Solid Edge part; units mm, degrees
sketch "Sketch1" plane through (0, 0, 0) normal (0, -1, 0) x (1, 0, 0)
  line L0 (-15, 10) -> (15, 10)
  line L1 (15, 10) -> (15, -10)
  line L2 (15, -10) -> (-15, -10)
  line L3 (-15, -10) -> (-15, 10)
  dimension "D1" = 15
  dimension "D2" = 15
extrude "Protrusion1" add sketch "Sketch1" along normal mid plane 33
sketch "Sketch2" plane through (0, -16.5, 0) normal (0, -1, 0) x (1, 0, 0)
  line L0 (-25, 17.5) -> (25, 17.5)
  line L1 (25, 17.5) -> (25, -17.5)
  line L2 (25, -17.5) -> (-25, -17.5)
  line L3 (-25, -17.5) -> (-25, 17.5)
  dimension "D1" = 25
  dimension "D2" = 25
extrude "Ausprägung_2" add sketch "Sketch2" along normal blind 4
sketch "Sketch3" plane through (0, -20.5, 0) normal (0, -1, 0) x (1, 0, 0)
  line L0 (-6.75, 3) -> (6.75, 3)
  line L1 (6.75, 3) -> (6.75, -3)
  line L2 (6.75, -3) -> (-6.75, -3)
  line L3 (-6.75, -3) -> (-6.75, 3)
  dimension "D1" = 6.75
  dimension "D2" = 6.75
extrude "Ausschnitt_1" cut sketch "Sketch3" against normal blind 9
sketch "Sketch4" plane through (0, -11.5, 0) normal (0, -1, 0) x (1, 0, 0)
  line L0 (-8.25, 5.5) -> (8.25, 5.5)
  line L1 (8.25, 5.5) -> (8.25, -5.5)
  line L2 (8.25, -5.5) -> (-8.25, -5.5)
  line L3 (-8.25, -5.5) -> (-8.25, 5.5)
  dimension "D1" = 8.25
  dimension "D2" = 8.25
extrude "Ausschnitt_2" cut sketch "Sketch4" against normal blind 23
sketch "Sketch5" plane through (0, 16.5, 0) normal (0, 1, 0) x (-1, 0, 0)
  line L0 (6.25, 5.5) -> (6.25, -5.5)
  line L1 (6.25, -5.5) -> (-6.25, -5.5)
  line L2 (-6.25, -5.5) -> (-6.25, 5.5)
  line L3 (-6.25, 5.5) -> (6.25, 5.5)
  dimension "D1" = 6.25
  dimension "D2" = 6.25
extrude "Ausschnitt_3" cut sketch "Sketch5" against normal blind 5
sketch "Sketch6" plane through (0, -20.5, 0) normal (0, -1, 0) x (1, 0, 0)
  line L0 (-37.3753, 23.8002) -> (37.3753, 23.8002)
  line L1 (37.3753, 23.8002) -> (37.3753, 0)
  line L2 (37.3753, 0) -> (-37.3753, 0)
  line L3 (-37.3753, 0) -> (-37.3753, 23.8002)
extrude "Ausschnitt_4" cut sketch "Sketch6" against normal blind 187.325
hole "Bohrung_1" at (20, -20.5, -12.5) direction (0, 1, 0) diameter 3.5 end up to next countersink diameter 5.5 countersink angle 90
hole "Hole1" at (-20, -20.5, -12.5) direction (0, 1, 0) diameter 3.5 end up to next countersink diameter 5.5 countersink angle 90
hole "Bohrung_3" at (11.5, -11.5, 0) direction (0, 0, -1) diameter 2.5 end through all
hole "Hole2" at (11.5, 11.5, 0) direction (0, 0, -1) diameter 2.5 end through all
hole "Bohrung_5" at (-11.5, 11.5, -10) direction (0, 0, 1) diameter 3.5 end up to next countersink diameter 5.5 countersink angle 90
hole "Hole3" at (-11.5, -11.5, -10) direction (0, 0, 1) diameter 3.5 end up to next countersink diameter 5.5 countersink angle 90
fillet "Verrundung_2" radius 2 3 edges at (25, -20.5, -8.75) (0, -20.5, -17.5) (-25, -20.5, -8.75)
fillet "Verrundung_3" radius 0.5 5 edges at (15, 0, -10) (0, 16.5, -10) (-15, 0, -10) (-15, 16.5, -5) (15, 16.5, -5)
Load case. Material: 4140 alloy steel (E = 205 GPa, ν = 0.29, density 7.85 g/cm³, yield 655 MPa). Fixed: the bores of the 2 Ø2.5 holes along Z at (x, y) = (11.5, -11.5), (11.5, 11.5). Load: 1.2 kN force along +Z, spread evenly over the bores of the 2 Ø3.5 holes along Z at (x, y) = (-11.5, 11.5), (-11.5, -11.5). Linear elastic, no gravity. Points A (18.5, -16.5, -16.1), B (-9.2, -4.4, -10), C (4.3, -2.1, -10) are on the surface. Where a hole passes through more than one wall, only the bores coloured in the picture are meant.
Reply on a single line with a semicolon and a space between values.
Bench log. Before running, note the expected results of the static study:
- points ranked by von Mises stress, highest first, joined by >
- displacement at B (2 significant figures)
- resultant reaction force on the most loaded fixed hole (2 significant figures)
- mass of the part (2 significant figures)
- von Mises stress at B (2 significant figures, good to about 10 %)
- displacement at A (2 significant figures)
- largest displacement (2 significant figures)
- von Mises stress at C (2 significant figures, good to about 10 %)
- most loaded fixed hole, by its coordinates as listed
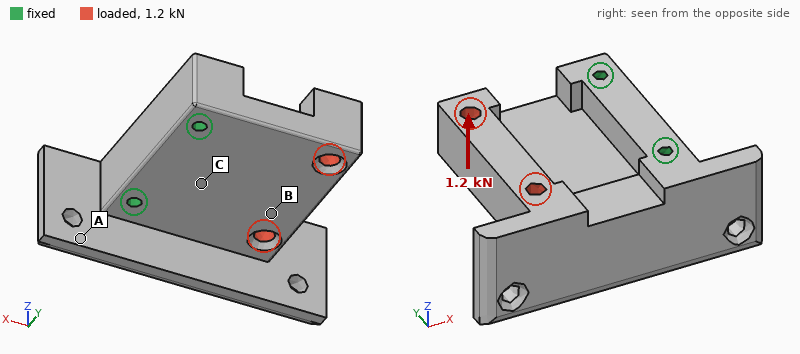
C > B > A; 32 µm; 630 N; 80 g; 32 MPa; 11 µm; 63 µm; 61 MPa; (11.5, -11.5)
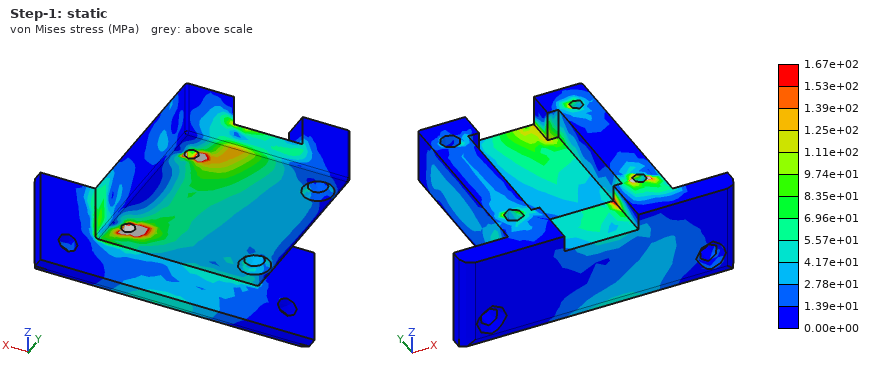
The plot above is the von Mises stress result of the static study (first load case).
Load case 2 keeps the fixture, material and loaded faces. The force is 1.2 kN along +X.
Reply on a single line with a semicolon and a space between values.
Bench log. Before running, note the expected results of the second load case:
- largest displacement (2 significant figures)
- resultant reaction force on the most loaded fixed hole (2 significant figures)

13 µm; 610 N
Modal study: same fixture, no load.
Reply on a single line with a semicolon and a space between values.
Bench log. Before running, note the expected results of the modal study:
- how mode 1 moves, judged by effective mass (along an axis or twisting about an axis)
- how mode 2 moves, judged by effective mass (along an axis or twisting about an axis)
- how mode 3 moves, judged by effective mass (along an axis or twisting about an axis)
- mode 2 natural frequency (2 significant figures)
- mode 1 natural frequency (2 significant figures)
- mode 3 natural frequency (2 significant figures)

along Z; twisting about X; along Y; 7900 Hz; 4800 Hz; 11 kHz
